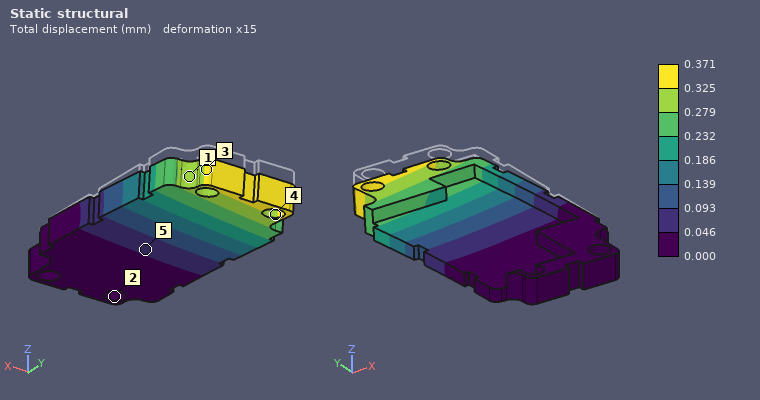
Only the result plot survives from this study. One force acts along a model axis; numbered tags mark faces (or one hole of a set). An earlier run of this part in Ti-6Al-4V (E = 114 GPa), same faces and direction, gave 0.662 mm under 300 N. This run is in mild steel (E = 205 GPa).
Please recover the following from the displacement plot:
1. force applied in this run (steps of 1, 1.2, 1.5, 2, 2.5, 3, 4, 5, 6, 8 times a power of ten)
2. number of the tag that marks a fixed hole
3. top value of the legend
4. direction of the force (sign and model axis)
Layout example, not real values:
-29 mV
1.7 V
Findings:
300 N
2
0.371 mm
-Z
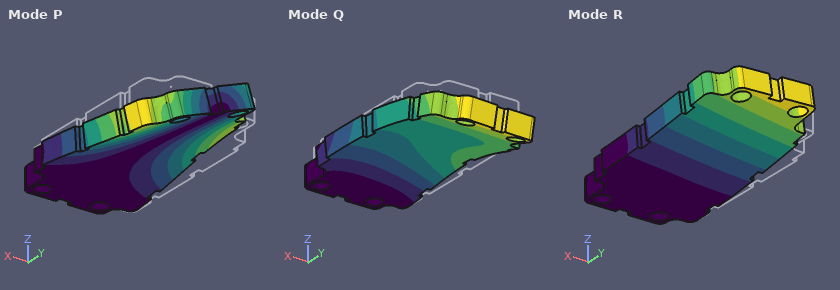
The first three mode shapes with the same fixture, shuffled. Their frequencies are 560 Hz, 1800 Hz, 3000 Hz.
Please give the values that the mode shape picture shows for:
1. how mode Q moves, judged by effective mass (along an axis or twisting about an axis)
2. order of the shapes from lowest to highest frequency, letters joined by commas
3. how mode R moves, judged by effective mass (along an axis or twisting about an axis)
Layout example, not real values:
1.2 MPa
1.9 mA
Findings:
along X
R, P, Q
along Z
